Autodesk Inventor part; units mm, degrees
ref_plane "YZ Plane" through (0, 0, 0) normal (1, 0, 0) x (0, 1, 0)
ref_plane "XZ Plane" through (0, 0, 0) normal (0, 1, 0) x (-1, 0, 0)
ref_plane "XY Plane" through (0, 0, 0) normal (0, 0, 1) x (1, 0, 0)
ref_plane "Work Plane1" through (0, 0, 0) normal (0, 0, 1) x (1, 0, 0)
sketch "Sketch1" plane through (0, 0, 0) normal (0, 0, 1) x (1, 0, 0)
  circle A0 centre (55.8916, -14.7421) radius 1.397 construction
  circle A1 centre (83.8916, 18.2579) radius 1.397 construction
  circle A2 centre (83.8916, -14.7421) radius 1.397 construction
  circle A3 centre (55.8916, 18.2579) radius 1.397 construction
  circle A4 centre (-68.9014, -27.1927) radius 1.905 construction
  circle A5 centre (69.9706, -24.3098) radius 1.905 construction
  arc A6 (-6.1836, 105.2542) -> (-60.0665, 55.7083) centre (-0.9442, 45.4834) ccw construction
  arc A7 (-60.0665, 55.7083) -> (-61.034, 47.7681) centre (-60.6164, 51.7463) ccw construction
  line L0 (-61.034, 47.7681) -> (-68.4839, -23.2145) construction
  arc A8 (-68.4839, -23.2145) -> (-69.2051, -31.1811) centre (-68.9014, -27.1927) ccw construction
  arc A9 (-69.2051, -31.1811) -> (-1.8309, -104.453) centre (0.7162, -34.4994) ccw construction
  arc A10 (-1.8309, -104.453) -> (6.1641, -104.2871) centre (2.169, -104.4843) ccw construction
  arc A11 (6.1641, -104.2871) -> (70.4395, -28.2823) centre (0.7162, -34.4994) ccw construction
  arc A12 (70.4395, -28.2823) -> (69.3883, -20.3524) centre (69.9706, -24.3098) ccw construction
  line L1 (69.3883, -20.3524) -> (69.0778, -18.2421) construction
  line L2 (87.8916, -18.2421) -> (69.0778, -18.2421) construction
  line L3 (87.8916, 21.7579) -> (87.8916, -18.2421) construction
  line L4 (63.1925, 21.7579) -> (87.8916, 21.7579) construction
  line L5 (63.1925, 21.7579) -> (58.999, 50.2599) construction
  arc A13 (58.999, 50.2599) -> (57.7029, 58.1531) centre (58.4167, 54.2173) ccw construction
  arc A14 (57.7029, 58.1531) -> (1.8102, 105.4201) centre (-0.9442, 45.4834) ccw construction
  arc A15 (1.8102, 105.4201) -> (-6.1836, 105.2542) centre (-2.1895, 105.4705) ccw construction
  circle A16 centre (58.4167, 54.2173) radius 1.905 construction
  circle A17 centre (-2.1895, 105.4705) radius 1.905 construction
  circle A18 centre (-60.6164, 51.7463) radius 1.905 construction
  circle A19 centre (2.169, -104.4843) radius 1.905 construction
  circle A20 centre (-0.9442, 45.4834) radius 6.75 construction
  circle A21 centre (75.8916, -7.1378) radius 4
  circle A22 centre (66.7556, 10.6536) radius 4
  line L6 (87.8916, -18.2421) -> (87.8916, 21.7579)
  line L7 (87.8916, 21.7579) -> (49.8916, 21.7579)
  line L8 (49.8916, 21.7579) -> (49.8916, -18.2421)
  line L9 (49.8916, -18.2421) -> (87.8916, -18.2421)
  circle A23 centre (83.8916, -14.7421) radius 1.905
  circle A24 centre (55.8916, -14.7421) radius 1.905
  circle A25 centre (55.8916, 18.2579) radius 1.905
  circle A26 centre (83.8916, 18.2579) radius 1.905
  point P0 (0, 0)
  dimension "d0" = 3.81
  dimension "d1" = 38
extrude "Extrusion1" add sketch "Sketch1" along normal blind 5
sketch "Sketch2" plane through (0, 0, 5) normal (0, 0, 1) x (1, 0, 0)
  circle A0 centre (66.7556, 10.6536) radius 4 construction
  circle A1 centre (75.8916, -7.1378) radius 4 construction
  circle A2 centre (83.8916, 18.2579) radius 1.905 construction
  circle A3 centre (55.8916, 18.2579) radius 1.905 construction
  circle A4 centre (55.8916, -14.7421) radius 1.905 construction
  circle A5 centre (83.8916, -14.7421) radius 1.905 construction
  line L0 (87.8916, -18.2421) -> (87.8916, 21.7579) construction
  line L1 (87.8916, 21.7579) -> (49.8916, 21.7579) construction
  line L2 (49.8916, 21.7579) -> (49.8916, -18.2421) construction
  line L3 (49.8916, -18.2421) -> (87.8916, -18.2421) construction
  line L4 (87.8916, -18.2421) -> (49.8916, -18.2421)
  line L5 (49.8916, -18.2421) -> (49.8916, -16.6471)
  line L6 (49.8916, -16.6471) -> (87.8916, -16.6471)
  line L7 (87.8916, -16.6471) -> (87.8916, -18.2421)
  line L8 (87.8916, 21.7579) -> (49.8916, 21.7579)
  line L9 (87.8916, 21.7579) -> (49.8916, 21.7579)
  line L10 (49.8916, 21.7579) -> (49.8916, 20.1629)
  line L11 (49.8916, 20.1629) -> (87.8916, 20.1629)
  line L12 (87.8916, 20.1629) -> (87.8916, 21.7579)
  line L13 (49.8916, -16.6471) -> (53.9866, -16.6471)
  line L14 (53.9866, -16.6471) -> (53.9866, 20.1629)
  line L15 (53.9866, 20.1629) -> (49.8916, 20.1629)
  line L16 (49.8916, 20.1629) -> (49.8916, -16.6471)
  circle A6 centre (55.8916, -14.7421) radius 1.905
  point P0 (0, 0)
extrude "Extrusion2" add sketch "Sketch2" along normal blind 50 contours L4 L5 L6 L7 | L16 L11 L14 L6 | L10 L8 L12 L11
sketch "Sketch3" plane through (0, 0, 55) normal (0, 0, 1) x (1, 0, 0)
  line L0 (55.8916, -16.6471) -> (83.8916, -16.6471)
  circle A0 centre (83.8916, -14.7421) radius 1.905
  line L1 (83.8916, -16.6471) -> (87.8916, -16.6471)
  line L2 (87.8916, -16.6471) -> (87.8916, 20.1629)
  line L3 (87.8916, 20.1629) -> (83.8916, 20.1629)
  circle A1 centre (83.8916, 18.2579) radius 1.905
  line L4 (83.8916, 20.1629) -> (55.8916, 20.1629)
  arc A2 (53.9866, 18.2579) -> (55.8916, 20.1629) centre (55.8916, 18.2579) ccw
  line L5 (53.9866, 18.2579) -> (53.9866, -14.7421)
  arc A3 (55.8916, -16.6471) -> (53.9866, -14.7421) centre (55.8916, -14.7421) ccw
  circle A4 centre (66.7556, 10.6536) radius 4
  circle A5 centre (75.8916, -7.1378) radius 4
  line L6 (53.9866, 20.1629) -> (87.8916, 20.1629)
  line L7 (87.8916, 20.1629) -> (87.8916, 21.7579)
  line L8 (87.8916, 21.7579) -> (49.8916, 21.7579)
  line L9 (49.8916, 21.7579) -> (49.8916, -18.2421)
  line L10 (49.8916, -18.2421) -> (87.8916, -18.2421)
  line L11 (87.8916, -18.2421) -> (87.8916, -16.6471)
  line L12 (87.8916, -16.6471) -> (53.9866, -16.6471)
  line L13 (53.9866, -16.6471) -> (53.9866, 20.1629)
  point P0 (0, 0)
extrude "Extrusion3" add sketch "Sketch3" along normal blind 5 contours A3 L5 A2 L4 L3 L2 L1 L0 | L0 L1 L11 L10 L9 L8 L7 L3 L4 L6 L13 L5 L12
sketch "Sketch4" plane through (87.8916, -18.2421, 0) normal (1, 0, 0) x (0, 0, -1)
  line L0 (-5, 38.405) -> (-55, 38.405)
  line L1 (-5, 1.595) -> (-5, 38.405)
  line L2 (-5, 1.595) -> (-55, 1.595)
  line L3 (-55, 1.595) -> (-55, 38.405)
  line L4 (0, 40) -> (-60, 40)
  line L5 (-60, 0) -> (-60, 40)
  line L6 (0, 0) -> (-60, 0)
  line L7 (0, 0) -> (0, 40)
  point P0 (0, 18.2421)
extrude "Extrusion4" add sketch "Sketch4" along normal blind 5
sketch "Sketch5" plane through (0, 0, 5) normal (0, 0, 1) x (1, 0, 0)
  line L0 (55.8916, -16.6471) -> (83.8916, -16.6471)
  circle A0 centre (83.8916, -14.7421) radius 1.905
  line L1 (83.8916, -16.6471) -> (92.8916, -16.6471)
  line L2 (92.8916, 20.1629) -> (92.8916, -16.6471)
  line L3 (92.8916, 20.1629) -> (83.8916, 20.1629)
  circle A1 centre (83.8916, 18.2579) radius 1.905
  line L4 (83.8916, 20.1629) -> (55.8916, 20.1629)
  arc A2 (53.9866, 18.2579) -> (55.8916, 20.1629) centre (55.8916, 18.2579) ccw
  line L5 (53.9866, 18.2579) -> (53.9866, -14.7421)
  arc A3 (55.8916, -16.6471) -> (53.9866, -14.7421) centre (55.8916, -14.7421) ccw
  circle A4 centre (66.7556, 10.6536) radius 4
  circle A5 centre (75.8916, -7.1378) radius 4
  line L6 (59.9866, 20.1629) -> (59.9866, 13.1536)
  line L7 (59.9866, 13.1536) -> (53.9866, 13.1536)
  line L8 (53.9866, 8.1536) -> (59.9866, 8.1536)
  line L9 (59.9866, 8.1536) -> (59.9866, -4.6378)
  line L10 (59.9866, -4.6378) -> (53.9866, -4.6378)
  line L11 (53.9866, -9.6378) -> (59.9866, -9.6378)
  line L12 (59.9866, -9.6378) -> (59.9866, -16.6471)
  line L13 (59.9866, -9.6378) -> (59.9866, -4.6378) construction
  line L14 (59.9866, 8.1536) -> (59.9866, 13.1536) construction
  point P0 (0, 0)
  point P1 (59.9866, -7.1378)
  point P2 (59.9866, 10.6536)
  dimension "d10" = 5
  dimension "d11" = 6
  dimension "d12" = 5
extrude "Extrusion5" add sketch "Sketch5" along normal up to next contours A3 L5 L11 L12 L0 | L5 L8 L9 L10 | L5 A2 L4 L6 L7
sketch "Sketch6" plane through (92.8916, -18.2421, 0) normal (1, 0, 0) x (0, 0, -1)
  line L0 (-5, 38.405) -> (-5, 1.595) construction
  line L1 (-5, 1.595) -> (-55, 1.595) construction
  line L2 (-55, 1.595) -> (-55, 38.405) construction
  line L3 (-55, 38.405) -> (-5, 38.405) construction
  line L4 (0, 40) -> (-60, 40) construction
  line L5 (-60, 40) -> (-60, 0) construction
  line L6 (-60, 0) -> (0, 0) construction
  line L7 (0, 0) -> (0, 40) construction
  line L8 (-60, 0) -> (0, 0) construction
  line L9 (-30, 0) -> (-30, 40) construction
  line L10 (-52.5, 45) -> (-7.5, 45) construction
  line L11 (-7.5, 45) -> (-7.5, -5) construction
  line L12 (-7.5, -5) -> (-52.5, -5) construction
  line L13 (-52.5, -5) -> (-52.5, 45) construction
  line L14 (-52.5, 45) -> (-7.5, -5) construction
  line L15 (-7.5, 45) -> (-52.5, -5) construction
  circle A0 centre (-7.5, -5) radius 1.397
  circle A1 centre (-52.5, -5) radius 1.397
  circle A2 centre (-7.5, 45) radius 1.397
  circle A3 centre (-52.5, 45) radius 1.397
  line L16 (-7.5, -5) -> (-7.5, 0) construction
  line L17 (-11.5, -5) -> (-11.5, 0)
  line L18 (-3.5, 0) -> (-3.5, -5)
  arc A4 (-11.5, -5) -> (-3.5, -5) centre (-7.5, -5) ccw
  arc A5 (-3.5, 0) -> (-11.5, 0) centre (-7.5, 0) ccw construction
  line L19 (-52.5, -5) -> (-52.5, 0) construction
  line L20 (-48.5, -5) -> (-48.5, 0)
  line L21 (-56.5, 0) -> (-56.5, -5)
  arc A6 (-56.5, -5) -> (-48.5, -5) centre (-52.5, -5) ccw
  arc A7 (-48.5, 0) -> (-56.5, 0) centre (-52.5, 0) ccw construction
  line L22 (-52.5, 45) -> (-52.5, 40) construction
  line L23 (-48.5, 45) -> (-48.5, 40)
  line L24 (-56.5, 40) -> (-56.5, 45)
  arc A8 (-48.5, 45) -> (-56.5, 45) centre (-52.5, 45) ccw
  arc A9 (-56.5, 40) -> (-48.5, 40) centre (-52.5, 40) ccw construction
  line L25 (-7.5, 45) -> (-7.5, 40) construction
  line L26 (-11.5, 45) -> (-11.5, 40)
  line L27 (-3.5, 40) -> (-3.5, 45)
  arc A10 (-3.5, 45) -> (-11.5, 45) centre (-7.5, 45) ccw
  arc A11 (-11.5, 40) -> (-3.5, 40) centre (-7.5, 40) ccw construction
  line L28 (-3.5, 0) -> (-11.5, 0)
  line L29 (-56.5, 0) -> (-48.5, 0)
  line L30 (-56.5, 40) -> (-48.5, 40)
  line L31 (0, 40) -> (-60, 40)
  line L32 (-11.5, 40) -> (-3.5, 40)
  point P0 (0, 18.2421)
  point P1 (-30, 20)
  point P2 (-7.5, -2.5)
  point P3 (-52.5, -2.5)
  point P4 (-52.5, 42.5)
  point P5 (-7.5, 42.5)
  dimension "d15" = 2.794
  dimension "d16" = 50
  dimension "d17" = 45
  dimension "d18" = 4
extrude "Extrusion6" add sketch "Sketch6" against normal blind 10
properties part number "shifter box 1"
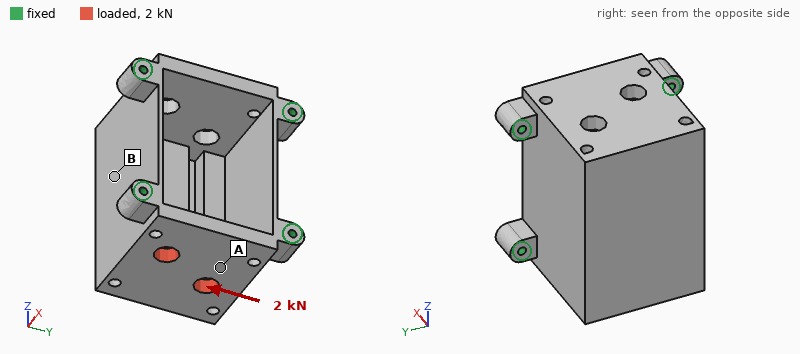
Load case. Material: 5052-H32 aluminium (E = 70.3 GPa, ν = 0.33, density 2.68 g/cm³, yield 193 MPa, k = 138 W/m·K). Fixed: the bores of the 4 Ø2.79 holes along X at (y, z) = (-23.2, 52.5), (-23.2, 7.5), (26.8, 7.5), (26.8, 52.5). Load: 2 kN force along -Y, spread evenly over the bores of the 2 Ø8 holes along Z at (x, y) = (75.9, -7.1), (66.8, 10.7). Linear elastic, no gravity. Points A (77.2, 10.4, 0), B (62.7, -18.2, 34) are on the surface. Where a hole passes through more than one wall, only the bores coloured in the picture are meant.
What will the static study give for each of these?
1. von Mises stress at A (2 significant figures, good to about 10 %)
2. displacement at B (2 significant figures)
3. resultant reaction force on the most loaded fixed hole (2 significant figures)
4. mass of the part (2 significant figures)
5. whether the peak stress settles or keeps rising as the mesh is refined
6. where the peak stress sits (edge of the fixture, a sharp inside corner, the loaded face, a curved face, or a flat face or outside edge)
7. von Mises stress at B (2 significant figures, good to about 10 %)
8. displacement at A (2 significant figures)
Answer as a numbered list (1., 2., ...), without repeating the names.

1. 19 MPa
2. 10 µm
3. 1.1 kN
4. 110 g
5. keeps rising
6. a sharp inside corner
7. 5.9 MPa
8. 11 µm
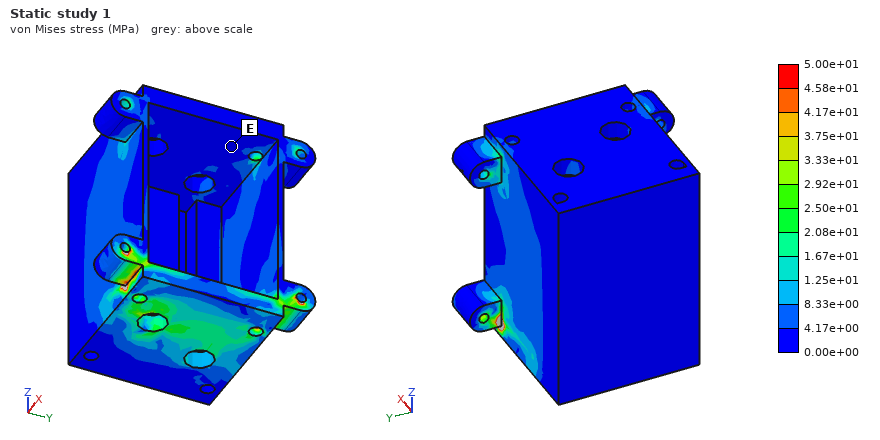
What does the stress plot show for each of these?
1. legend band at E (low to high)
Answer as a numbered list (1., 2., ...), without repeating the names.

1. 0.00e+00 to 4.17e+00 MPa
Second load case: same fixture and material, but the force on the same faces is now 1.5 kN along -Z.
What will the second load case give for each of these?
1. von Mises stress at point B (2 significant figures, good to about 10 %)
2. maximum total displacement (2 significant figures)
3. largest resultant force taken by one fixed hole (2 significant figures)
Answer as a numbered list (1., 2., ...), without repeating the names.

1. 7.1 MPa
2. 30 µm
3. 670 N
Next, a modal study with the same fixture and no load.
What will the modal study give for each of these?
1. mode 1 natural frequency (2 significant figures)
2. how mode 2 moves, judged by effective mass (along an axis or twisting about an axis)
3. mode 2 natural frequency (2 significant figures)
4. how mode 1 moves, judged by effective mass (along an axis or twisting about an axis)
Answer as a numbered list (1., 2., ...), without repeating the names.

1. 5200 Hz
2. along Y
3. 5600 Hz
4. along Z
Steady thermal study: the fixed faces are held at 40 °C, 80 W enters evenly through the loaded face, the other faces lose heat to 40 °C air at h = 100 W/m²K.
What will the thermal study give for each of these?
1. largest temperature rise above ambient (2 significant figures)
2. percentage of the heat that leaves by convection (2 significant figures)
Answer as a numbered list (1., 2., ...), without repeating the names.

1. 48 K
2. 45 %
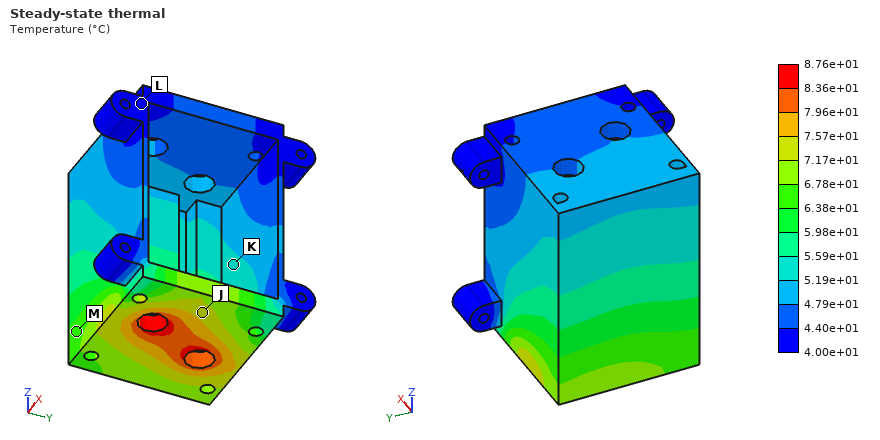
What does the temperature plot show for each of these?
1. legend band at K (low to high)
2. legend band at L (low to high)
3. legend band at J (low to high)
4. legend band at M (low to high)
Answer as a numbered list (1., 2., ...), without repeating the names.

1. 5.19e+01 to 5.59e+01 °C
2. 4.00e+01 to 4.40e+01 °C
3. 7.17e+01 to 7.57e+01 °C
4. 6.38e+01 to 6.78e+01 °C
